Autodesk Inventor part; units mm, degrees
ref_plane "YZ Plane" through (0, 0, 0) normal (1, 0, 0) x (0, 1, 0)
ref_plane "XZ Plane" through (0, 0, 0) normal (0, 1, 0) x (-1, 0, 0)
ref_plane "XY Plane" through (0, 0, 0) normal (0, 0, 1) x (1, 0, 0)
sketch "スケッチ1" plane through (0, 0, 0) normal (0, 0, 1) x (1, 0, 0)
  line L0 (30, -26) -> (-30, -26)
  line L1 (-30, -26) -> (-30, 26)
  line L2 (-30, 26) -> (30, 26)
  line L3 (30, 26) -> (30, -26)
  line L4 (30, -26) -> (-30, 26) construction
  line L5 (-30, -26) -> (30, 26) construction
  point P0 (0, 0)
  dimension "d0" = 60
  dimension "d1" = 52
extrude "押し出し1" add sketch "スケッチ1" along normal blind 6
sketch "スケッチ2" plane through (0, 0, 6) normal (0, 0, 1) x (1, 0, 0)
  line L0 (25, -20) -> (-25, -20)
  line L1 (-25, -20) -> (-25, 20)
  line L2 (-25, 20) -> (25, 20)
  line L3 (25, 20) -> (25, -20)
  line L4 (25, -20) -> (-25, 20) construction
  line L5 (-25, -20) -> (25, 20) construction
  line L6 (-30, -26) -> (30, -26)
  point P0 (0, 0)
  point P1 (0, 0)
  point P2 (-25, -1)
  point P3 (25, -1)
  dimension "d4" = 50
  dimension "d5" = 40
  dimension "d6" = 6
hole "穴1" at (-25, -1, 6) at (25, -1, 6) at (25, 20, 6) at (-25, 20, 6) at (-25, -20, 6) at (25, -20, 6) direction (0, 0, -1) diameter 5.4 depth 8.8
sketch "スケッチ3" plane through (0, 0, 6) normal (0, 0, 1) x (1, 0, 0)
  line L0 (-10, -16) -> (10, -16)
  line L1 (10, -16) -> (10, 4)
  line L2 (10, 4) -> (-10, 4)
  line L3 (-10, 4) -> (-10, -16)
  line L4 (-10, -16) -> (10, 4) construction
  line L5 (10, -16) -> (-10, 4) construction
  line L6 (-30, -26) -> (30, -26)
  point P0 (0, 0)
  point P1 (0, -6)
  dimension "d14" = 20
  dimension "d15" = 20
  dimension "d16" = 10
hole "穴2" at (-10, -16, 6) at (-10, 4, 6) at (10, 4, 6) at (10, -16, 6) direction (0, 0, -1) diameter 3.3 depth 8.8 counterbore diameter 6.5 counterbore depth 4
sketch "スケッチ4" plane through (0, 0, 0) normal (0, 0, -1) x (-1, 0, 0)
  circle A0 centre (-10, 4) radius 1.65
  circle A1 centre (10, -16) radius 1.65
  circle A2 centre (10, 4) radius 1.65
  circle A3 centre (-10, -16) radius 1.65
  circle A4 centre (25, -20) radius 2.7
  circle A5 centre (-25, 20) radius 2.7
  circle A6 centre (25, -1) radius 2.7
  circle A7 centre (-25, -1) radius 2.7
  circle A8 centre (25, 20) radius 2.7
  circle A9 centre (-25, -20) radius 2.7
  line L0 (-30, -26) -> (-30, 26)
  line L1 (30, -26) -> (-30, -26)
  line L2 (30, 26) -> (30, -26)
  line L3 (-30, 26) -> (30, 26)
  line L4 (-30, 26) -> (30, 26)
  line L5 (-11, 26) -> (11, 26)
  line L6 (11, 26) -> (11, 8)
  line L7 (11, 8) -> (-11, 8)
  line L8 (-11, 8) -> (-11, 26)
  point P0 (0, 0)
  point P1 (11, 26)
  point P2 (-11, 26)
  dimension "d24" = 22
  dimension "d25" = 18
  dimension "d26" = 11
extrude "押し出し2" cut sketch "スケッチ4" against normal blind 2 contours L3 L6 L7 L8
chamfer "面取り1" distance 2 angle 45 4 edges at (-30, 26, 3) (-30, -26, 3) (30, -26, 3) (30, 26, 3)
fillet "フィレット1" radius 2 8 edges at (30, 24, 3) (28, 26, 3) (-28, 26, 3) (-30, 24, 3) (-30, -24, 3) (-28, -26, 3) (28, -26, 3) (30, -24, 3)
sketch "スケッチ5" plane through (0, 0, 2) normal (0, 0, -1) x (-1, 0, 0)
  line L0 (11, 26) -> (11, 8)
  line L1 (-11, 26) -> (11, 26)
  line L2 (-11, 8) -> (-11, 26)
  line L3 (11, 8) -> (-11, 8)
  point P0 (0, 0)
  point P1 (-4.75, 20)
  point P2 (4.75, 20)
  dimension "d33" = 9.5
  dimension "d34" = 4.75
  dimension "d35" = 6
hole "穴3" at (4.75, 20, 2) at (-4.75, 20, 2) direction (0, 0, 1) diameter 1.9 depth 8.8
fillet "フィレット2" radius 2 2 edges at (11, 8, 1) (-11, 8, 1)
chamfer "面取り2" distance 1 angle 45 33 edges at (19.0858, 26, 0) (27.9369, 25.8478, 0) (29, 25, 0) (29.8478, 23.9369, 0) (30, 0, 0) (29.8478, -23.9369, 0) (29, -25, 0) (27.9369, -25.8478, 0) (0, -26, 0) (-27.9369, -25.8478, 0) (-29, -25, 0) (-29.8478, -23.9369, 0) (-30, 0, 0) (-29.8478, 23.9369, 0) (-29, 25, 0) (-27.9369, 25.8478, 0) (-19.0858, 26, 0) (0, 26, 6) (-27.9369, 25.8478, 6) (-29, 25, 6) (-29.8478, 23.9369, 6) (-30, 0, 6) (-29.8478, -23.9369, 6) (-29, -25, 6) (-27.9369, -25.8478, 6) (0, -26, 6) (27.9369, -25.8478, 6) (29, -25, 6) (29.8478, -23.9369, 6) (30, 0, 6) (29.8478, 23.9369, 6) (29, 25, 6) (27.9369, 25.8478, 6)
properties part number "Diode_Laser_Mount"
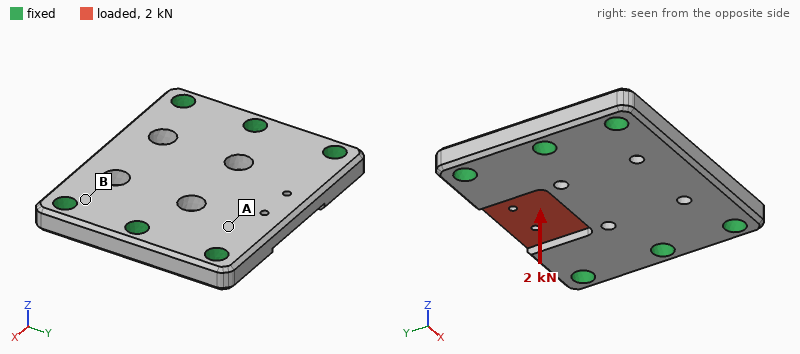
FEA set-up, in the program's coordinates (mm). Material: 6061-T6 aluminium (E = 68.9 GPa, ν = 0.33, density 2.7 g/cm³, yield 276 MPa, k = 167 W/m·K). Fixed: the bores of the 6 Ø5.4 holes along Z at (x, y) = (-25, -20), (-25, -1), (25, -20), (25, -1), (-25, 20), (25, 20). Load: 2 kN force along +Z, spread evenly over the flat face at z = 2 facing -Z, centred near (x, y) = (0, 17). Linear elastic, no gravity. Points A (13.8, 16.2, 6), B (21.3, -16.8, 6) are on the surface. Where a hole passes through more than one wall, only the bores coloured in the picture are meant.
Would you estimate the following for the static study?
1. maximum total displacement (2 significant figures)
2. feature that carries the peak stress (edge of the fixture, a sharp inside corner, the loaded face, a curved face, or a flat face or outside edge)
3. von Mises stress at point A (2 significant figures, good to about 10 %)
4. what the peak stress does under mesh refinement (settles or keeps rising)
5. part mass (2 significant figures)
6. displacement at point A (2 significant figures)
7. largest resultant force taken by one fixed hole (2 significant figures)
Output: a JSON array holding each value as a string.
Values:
["70 µm", "edge of the fixture", "31 MPa", "keeps rising", "44 g", "21 µm", "940 N"]
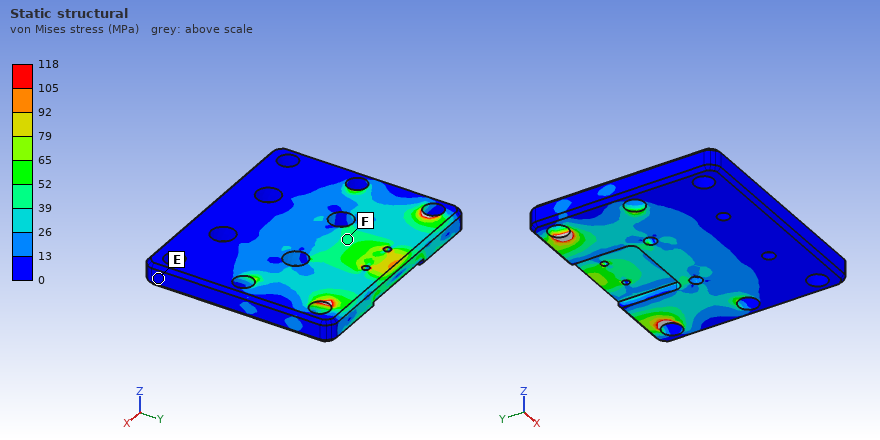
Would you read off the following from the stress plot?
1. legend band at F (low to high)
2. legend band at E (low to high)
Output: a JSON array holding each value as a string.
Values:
["39 to 52 MPa", "0 to 13 MPa"]
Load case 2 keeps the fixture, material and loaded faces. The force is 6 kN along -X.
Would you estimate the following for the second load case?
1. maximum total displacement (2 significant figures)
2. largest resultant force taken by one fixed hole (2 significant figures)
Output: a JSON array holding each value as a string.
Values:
["14 µm", "2.0 kN"]
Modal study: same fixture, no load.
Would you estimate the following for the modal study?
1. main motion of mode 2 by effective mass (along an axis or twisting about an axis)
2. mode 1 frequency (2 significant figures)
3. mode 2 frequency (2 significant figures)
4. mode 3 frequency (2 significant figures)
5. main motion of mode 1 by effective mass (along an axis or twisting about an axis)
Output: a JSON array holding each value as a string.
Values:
["twisting about X", "12 kHz", "14 kHz", "21 kHz", "along Z"]
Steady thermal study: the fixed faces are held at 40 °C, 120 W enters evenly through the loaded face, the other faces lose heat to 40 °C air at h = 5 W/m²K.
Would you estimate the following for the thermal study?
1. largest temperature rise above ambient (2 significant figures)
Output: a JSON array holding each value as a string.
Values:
["58 K"]
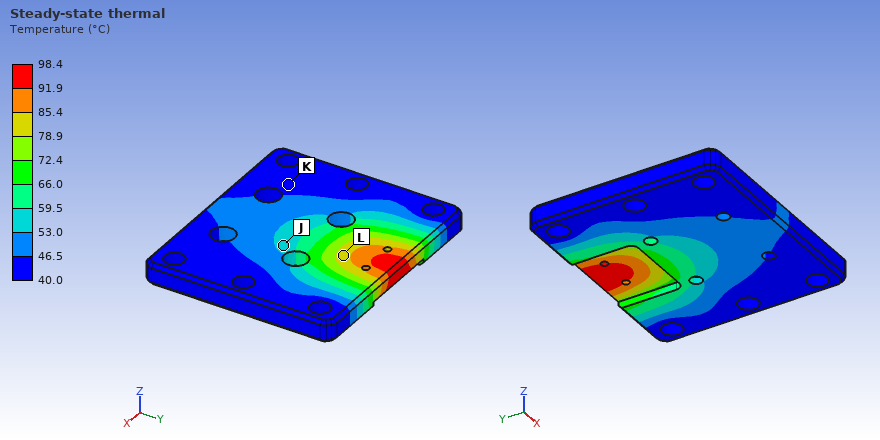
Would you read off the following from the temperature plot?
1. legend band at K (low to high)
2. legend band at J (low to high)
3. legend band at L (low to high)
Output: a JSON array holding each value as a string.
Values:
["40.0 to 46.5 °C", "53.0 to 59.5 °C", "78.9 to 85.4 °C"]
